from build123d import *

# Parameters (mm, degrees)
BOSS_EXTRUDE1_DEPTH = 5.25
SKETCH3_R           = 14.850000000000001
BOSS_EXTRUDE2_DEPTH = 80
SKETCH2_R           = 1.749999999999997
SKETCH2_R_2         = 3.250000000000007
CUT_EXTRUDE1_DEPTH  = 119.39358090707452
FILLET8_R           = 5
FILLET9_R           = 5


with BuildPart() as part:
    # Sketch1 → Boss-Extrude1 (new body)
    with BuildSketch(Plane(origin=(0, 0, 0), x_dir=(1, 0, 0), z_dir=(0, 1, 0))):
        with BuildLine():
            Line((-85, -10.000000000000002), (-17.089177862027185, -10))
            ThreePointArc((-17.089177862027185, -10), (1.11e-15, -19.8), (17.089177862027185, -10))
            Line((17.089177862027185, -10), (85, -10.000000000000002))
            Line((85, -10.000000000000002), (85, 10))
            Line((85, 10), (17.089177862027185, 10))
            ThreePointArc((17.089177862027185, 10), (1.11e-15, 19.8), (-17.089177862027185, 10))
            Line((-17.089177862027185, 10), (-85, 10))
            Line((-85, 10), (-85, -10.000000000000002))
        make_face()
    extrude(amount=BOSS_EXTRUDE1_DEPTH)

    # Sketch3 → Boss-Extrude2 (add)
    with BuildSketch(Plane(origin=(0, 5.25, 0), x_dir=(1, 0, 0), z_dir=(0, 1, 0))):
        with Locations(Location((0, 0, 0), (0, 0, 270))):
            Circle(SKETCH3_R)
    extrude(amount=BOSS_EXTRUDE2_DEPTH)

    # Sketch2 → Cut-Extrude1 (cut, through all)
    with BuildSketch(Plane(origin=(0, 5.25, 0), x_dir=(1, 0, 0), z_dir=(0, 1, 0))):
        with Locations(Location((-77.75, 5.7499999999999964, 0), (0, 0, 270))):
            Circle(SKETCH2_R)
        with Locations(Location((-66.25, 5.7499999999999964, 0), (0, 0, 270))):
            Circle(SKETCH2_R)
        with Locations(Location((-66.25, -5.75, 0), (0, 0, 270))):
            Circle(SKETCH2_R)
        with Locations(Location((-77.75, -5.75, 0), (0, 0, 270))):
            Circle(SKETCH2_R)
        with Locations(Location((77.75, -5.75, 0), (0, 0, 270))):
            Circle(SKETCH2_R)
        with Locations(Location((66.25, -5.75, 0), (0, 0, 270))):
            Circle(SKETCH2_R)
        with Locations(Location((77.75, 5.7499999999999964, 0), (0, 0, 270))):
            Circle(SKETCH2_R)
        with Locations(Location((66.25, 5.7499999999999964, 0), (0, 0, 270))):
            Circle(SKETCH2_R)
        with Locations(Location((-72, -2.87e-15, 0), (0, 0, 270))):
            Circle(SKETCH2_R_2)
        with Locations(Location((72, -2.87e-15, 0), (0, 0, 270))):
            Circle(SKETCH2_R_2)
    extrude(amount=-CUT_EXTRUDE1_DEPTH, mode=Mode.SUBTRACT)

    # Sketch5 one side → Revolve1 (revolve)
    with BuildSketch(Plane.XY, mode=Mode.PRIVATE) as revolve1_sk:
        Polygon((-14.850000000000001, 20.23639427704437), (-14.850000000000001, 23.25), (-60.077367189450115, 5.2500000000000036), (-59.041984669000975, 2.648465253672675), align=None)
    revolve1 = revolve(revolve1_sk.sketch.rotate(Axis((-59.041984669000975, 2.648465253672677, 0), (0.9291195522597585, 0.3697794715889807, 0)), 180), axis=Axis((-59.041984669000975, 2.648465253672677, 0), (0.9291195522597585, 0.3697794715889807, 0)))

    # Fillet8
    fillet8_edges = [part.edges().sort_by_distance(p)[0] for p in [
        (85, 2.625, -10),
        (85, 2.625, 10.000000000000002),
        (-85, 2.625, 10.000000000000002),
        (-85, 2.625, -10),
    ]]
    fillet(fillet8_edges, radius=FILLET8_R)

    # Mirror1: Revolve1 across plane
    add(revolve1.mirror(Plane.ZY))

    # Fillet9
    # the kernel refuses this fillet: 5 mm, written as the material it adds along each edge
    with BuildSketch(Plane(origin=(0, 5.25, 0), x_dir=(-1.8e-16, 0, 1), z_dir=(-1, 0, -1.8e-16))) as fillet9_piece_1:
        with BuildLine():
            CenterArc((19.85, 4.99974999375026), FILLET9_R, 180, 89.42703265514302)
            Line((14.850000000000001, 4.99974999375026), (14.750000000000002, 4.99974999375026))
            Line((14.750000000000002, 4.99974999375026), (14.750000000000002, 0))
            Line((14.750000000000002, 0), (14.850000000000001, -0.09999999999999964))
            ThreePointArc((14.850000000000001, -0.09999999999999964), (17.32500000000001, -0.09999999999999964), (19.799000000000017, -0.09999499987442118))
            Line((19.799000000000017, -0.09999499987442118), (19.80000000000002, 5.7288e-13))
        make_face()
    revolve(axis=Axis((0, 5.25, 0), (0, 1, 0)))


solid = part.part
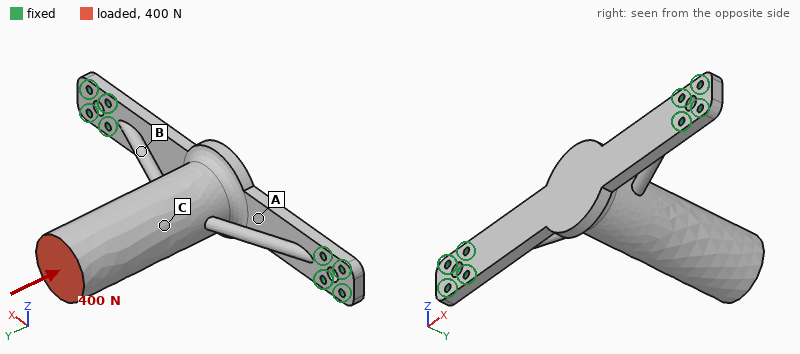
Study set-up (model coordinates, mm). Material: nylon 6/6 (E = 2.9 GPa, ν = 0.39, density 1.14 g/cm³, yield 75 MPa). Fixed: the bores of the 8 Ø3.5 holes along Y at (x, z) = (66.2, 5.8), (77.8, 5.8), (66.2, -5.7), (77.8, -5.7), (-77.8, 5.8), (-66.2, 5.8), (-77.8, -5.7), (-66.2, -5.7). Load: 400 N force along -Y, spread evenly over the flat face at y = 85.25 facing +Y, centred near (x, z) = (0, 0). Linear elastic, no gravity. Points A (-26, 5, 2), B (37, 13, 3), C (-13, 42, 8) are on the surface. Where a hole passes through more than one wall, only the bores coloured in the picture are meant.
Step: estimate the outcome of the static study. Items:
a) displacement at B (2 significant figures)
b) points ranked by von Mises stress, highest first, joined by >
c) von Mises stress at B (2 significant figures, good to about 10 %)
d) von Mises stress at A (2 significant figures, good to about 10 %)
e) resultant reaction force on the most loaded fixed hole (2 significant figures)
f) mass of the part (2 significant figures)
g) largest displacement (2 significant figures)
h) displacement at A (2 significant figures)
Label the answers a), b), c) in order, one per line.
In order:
a) 0.48 mm
b) B > A > C
c) 17 MPa
d) 5.4 MPa
e) 190 N
f) 88 g
g) 0.80 mm
h) 0.68 mm
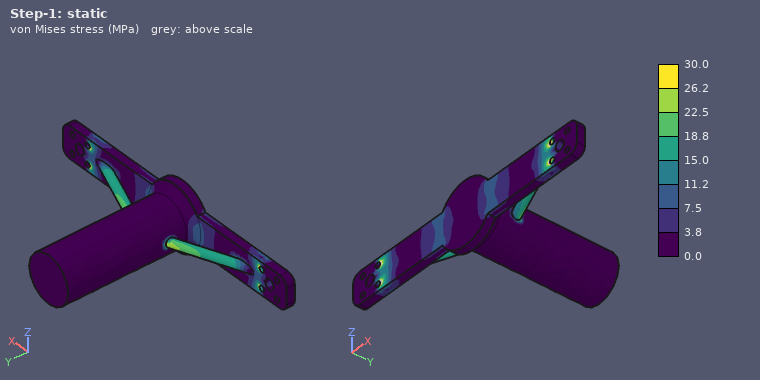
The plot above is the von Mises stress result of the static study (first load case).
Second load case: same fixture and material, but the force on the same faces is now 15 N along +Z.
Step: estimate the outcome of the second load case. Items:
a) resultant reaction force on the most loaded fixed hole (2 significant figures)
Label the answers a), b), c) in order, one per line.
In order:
a) 46 N
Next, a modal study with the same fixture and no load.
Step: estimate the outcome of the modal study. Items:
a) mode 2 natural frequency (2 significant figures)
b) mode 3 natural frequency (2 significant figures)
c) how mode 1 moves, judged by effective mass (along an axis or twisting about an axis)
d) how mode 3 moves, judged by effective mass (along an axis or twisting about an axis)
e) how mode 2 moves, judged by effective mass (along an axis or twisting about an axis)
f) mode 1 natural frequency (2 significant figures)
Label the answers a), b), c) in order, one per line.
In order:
a) 410 Hz
b) 480 Hz
c) along Z
d) along X
e) along Y
f) 87 Hz
